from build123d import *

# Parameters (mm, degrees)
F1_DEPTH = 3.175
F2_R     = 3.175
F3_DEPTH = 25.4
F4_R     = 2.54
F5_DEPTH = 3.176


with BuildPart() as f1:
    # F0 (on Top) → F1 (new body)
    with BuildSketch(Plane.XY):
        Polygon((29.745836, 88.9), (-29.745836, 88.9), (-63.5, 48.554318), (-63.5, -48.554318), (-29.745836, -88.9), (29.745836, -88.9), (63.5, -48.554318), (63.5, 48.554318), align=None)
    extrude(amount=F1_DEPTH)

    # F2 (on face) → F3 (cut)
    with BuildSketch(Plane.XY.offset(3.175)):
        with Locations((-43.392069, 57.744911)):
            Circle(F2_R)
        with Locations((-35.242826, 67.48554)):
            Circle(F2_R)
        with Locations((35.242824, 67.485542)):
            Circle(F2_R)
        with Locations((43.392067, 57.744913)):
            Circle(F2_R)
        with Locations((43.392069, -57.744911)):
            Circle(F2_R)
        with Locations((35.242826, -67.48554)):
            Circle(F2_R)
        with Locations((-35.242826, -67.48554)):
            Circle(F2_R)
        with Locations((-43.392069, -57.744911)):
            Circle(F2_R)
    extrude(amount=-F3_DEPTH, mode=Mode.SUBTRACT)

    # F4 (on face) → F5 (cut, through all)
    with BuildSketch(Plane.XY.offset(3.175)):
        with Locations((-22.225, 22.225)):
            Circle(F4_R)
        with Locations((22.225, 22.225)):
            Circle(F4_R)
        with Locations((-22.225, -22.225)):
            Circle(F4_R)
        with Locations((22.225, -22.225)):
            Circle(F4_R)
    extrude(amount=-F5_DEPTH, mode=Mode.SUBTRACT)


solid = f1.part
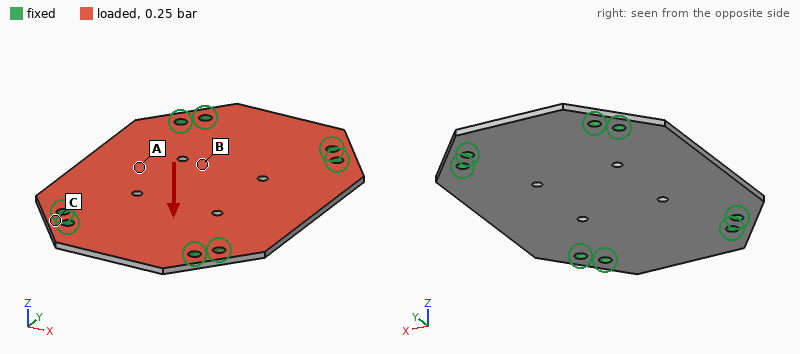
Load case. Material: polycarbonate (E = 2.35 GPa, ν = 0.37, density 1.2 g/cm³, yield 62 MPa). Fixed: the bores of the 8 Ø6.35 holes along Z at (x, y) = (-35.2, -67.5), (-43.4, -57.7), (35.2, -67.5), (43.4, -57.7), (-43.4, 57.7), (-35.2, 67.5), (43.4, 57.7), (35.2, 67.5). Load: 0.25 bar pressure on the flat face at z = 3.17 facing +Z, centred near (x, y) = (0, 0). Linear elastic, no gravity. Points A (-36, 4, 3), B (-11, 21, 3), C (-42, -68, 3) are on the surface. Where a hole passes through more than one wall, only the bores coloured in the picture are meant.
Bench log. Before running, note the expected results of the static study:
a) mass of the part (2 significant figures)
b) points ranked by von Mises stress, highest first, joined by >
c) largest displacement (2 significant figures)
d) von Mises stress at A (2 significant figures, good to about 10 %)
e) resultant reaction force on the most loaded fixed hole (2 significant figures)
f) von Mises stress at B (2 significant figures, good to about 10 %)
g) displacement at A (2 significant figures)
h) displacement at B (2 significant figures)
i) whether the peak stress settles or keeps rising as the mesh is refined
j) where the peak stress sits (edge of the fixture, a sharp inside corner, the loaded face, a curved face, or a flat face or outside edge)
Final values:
74 g
A > B > C
2.4 mm
8.3 MPa
94 N
5.8 MPa
2.2 mm
2.0 mm
keeps rising
edge of the fixture
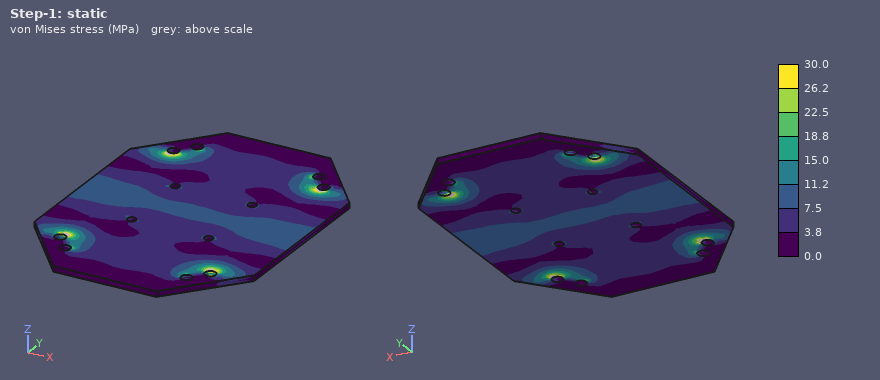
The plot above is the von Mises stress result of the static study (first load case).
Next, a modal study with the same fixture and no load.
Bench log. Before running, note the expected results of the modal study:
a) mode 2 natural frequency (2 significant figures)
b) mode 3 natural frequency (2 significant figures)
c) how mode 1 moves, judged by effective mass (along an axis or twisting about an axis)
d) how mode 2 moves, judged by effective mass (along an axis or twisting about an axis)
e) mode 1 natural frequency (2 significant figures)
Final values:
390 Hz
520 Hz
along Z
twisting about Y
310 Hz
